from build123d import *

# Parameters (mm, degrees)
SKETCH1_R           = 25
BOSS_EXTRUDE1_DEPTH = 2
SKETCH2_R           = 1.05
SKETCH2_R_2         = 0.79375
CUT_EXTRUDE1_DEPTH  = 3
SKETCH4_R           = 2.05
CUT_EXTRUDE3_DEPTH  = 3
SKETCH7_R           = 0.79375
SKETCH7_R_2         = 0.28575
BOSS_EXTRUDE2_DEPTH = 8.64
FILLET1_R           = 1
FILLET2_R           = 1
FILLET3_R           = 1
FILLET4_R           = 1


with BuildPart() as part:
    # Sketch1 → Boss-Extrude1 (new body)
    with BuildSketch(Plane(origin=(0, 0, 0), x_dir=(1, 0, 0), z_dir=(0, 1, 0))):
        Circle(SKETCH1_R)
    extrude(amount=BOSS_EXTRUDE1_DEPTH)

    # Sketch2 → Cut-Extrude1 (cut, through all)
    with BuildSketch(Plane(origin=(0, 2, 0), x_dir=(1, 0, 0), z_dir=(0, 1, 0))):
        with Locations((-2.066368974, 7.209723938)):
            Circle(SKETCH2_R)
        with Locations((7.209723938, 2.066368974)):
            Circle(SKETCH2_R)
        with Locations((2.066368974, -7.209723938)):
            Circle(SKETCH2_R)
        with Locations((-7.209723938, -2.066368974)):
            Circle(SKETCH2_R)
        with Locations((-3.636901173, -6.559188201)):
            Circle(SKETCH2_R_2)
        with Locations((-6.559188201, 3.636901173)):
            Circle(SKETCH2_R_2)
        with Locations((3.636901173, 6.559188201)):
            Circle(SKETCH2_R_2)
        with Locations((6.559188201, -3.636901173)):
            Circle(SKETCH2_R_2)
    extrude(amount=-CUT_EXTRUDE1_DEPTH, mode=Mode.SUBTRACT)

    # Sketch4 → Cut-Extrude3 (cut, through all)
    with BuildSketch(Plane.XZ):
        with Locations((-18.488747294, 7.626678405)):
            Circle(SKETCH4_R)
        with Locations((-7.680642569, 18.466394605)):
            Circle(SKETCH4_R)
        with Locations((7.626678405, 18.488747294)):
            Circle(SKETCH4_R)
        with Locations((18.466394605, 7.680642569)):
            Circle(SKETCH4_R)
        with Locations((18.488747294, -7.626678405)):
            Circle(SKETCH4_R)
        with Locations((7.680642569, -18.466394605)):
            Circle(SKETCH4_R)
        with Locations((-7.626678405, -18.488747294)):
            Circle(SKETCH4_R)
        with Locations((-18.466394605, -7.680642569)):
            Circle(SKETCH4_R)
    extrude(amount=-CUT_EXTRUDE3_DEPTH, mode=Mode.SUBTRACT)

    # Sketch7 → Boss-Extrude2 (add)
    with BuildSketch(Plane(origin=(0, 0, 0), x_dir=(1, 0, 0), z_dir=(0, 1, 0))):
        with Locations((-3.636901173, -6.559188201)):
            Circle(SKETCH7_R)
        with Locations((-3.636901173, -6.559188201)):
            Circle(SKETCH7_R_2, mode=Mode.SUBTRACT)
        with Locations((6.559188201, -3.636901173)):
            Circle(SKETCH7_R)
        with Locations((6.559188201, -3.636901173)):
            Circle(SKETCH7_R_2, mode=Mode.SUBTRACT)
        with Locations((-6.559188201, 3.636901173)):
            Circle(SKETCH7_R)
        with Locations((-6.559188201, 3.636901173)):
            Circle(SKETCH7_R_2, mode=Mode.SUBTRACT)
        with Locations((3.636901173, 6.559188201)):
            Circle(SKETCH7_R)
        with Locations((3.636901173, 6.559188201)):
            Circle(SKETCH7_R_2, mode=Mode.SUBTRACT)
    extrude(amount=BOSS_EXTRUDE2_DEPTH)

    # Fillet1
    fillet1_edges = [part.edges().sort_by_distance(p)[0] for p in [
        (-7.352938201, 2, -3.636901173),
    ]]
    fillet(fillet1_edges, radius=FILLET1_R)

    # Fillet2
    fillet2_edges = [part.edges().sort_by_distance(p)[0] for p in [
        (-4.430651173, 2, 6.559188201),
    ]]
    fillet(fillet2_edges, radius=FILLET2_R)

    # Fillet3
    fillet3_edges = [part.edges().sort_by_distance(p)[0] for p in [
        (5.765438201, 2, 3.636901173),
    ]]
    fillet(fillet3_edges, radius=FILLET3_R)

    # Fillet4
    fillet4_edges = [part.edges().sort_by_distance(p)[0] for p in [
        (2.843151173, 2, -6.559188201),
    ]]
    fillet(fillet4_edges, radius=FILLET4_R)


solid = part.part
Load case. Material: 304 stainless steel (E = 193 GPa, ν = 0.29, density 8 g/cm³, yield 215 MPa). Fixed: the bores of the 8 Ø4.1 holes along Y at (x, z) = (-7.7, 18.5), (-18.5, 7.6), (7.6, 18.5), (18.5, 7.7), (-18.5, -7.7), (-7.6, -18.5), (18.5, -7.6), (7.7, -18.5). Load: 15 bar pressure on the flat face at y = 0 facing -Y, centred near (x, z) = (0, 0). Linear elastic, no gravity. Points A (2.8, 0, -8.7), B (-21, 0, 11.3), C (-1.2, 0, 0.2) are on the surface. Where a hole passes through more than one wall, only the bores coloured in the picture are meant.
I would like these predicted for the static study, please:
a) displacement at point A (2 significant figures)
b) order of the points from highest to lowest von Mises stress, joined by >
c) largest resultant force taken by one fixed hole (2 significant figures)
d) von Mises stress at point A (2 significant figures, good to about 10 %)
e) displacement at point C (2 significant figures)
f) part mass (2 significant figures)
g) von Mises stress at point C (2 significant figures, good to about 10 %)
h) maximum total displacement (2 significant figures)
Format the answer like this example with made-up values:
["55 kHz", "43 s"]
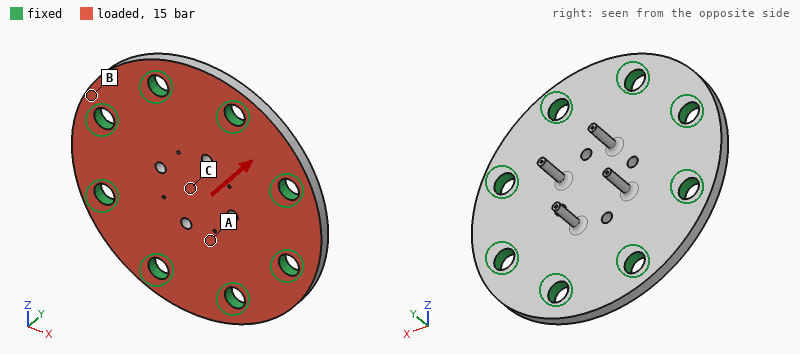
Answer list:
["14 µm", "C > A > B", "350 N", "34 MPa", "23 µm", "30 g", "62 MPa", "23 µm"]
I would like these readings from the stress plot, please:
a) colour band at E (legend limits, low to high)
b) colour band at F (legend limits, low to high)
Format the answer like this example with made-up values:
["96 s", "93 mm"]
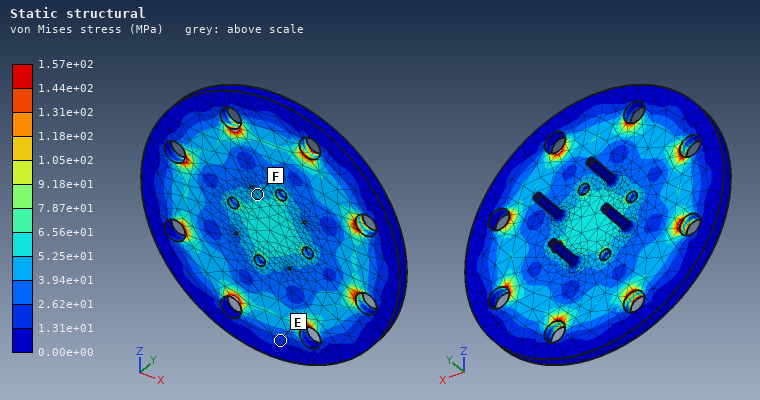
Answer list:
["1.31e+01 to 2.62e+01 MPa", "3.94e+01 to 5.25e+01 MPa"]
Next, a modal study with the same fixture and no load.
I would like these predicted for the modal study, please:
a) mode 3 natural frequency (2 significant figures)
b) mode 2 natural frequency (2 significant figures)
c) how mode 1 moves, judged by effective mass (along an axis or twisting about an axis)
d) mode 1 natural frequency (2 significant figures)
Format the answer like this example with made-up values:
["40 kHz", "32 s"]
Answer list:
["24 kHz", "24 kHz", "along Y", "12 kHz"]
